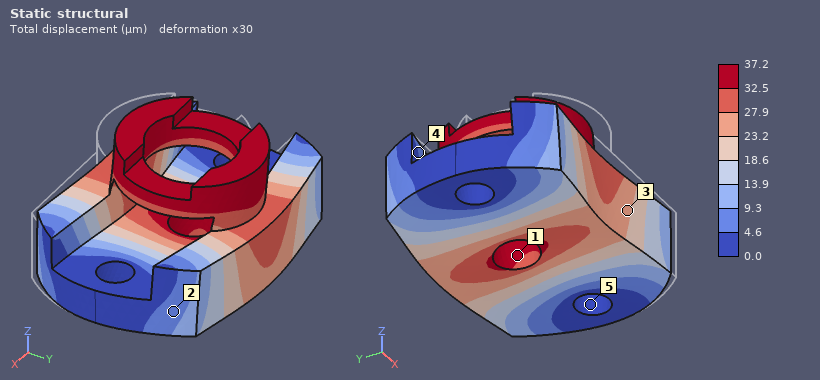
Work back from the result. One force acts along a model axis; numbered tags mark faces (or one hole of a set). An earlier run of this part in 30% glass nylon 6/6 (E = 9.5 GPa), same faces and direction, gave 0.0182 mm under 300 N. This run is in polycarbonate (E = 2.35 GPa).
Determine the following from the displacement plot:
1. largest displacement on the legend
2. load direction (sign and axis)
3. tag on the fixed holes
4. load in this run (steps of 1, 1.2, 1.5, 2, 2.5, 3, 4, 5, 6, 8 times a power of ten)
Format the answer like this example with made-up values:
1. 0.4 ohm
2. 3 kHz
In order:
1. 37.2 µm
2. +Y
3. 5
4. 150 N
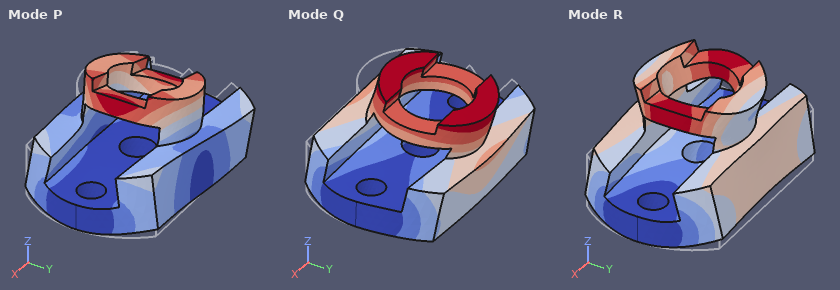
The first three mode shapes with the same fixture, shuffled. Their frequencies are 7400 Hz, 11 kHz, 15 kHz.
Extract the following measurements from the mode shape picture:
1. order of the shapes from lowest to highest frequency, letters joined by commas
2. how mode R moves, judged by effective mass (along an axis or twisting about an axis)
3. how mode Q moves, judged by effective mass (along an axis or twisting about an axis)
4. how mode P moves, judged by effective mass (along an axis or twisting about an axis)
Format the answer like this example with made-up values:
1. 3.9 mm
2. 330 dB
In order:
1. Q, R, P
2. along Z
3. along Y
4. along X
